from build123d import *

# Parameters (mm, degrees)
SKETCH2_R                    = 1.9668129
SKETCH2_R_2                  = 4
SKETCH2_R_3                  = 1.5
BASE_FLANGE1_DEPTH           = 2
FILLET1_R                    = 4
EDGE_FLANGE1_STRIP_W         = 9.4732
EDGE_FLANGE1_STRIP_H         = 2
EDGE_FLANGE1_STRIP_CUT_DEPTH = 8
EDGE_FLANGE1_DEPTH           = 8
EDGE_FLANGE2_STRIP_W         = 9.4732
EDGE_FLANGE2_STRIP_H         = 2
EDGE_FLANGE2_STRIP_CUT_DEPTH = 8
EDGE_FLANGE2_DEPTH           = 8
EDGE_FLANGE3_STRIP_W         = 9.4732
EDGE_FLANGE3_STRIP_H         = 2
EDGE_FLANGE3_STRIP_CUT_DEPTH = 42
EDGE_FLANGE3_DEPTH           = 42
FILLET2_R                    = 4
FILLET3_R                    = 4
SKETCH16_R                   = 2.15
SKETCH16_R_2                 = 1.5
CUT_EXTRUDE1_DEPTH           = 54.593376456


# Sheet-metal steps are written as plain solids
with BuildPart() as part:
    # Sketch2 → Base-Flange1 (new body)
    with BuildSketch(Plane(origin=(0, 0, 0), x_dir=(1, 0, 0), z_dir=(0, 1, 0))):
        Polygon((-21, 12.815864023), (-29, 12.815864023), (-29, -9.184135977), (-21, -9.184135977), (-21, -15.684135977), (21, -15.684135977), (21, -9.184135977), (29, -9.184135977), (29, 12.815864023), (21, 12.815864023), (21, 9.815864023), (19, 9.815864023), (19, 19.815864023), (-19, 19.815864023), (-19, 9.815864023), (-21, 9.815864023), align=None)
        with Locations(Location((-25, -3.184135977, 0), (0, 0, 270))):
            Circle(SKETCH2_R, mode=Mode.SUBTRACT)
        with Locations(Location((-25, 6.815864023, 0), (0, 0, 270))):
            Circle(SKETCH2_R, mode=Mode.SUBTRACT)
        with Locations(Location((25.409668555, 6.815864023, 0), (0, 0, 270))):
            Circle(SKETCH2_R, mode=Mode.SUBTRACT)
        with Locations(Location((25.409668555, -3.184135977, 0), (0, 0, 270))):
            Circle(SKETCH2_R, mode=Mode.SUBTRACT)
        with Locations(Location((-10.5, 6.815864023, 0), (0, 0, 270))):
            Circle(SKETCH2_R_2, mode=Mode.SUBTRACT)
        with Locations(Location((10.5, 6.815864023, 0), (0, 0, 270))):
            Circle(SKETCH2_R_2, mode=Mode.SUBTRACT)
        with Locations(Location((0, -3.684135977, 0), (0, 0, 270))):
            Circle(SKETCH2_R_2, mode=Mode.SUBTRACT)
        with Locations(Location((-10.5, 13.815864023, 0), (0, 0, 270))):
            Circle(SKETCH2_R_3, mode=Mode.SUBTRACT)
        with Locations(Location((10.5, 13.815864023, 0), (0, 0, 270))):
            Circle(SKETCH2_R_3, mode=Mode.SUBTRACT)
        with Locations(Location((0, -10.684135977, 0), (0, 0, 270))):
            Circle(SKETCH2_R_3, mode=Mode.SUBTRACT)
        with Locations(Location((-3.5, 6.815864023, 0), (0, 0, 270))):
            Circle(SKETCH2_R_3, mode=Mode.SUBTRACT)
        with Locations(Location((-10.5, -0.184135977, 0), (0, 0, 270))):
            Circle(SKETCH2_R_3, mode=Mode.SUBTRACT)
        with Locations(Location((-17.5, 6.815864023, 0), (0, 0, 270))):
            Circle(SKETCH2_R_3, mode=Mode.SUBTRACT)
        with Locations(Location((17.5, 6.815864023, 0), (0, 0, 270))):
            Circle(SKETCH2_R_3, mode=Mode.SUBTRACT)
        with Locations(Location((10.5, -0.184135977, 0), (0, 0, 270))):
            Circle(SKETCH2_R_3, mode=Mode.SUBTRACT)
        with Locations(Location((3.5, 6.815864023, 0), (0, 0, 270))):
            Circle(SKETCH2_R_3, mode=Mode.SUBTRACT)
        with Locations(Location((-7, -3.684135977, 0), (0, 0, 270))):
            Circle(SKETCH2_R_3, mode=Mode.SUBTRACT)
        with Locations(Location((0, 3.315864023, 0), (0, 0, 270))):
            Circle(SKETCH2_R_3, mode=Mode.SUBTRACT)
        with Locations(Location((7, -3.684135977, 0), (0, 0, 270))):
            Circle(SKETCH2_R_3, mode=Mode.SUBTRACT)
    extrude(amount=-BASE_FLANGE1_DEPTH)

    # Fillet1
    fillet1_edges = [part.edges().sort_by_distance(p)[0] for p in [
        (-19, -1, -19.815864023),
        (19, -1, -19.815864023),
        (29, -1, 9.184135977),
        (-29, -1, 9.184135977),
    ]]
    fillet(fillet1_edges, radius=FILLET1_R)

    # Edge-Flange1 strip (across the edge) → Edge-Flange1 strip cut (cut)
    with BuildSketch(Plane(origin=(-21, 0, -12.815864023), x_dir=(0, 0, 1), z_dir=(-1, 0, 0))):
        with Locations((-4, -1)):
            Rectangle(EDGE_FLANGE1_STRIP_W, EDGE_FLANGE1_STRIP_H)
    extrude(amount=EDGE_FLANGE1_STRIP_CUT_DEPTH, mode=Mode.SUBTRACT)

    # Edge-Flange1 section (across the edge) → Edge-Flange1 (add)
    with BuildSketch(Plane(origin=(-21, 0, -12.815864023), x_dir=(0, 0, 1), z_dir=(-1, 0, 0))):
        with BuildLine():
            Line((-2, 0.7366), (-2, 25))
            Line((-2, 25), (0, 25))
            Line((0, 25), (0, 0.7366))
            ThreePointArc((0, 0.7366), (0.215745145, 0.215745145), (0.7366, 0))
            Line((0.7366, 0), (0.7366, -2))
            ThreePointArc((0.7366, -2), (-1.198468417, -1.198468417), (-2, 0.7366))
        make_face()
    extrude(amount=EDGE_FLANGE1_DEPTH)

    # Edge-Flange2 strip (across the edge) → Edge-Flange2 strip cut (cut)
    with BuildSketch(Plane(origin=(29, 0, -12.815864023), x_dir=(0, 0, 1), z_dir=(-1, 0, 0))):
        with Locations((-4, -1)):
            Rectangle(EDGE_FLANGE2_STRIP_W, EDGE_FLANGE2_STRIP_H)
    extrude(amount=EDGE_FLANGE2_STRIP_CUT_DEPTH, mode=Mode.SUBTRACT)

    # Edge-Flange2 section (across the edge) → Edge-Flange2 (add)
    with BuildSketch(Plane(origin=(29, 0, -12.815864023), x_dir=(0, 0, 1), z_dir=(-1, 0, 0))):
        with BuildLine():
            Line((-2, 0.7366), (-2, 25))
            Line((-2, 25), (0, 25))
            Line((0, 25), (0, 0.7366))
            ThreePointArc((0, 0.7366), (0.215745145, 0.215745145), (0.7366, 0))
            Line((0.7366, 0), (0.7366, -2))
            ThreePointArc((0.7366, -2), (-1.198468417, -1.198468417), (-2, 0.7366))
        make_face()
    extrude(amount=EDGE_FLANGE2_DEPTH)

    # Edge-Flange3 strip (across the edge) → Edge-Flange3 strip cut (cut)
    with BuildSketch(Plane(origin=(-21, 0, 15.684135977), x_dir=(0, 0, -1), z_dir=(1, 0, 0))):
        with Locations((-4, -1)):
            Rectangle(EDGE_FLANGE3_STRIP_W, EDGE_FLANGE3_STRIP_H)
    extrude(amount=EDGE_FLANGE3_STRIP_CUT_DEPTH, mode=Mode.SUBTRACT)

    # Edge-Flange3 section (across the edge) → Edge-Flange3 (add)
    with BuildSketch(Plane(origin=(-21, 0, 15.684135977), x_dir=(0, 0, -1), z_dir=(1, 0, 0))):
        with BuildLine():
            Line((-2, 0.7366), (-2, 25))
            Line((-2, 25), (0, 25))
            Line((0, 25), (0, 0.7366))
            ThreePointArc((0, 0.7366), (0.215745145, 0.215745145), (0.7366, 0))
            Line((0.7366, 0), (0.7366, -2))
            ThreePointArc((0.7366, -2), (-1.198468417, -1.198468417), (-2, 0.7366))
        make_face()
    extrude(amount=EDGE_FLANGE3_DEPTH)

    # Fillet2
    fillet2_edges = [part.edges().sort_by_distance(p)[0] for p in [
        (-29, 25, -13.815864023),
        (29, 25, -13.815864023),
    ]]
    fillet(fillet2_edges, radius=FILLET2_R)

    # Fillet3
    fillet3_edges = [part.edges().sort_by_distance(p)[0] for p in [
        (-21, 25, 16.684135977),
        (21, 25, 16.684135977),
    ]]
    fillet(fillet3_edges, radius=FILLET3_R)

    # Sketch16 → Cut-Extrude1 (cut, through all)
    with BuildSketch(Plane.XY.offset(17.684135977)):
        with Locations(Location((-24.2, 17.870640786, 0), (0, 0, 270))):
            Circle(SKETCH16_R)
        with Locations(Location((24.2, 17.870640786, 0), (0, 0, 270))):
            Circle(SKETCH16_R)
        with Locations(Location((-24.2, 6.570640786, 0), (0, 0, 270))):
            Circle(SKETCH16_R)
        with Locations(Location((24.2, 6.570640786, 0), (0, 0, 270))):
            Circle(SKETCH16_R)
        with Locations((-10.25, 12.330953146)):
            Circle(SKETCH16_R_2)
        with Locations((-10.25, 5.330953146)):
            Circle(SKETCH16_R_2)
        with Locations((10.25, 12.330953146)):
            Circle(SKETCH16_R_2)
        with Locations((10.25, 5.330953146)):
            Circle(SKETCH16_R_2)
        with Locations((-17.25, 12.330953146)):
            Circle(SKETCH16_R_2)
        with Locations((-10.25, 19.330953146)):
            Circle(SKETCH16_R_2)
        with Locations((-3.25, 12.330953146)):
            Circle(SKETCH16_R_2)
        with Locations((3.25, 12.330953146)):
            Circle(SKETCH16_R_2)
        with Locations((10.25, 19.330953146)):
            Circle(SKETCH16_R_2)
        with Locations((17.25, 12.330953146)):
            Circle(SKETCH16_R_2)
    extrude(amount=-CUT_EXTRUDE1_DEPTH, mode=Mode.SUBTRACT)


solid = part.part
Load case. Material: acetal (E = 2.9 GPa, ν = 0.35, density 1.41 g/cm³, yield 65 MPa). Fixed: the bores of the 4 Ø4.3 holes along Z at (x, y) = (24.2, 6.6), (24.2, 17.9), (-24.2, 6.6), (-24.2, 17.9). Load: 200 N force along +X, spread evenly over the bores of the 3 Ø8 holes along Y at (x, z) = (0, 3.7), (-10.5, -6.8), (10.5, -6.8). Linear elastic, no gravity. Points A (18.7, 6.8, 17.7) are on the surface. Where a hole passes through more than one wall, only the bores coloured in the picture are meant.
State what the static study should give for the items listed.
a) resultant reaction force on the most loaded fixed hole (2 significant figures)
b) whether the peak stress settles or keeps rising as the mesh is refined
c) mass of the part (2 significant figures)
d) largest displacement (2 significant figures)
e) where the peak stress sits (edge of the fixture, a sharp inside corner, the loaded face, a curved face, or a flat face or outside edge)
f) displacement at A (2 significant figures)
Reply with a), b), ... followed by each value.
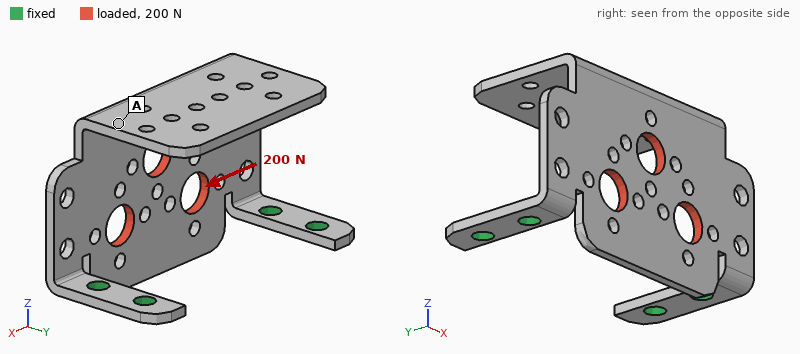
a) 120 N
b) keeps rising
c) 8.1 g
d) 0.87 mm
e) edge of the fixture
f) 0.62 mm
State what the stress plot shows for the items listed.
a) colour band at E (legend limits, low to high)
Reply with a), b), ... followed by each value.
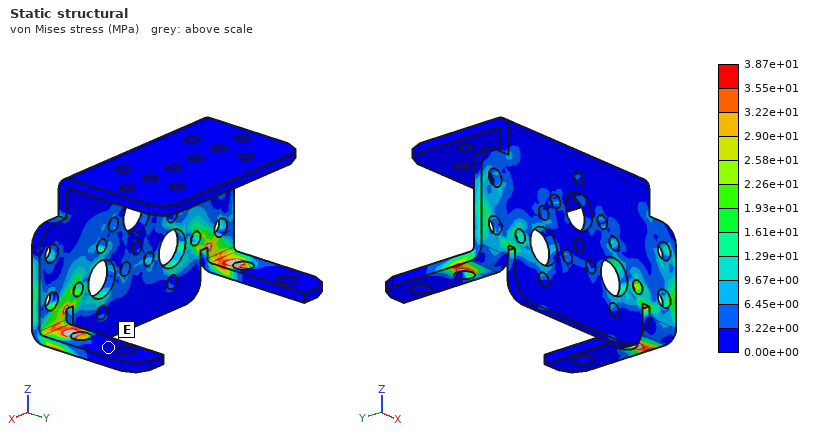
a) 0.00e+00 to 3.22e+00 MPa
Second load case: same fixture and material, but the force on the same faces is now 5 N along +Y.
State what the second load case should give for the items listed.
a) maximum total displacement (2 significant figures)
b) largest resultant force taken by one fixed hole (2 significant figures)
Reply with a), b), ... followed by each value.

a) 0.77 mm
b) 2.6 N
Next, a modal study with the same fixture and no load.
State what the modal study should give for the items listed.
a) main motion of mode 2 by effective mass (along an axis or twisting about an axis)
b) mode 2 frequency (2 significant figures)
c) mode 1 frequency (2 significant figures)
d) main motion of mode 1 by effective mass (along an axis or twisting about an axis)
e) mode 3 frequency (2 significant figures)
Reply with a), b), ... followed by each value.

a) along X
b) 330 Hz
c) 110 Hz
d) along Y
e) 430 Hz
